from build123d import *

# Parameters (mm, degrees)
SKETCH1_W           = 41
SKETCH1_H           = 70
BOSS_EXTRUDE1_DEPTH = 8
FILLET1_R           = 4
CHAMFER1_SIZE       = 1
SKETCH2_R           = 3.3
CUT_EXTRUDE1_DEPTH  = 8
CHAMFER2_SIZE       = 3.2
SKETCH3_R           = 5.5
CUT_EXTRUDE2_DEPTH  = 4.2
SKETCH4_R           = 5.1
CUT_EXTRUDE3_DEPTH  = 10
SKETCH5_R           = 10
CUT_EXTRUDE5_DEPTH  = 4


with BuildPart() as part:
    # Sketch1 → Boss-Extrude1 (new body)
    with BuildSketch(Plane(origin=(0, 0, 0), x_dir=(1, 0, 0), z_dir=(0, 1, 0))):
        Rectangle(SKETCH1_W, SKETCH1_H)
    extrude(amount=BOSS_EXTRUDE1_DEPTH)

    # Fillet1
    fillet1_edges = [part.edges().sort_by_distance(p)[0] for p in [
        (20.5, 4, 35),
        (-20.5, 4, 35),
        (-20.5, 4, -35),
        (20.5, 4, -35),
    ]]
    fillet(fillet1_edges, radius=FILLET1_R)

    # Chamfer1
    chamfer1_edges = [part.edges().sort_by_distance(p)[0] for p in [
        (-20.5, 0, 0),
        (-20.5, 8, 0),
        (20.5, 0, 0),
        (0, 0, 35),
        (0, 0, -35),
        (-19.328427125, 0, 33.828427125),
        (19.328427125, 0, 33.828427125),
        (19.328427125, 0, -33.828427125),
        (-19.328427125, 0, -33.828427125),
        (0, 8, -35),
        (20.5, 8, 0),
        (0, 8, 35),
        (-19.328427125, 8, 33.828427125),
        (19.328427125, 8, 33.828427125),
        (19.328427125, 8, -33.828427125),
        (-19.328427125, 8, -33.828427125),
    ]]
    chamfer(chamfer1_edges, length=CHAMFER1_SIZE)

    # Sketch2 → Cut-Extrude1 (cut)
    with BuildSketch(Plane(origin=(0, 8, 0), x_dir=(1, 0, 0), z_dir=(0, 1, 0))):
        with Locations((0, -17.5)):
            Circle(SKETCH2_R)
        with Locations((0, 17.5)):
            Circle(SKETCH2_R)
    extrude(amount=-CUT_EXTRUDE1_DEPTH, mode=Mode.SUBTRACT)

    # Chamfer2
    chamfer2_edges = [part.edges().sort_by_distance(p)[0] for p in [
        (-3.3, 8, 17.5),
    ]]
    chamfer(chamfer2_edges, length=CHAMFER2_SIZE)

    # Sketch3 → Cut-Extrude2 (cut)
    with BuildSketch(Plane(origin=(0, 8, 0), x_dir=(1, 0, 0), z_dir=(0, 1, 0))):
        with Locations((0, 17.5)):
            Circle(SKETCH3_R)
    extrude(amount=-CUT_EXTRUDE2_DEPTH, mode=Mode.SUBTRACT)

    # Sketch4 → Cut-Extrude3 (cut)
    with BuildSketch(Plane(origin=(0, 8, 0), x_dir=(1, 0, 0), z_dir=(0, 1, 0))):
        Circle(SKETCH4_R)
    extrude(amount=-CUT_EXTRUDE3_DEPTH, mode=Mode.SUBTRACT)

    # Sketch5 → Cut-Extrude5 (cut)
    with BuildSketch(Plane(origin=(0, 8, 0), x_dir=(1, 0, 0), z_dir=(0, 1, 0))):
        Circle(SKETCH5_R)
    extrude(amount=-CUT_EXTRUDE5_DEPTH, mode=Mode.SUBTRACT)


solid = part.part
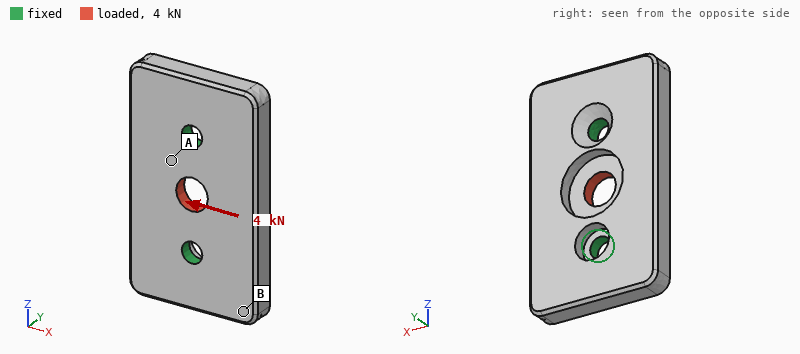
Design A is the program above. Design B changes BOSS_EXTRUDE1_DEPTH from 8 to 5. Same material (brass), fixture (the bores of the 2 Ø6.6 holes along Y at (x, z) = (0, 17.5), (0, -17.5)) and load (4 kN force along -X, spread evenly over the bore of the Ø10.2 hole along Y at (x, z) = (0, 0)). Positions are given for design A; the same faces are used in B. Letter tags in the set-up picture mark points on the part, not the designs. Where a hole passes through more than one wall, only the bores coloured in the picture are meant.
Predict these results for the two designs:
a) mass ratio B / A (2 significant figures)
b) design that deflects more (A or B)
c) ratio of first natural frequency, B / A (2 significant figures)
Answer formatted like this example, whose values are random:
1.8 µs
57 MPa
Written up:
0.64
B
0.79
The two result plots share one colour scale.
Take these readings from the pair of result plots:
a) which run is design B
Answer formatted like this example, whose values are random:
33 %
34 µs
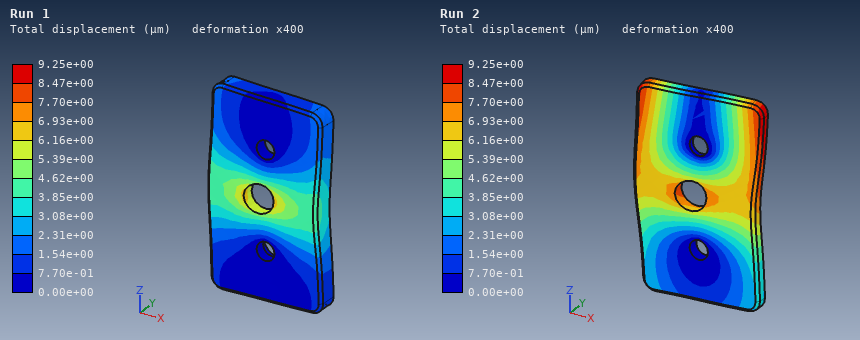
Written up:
Run 2
